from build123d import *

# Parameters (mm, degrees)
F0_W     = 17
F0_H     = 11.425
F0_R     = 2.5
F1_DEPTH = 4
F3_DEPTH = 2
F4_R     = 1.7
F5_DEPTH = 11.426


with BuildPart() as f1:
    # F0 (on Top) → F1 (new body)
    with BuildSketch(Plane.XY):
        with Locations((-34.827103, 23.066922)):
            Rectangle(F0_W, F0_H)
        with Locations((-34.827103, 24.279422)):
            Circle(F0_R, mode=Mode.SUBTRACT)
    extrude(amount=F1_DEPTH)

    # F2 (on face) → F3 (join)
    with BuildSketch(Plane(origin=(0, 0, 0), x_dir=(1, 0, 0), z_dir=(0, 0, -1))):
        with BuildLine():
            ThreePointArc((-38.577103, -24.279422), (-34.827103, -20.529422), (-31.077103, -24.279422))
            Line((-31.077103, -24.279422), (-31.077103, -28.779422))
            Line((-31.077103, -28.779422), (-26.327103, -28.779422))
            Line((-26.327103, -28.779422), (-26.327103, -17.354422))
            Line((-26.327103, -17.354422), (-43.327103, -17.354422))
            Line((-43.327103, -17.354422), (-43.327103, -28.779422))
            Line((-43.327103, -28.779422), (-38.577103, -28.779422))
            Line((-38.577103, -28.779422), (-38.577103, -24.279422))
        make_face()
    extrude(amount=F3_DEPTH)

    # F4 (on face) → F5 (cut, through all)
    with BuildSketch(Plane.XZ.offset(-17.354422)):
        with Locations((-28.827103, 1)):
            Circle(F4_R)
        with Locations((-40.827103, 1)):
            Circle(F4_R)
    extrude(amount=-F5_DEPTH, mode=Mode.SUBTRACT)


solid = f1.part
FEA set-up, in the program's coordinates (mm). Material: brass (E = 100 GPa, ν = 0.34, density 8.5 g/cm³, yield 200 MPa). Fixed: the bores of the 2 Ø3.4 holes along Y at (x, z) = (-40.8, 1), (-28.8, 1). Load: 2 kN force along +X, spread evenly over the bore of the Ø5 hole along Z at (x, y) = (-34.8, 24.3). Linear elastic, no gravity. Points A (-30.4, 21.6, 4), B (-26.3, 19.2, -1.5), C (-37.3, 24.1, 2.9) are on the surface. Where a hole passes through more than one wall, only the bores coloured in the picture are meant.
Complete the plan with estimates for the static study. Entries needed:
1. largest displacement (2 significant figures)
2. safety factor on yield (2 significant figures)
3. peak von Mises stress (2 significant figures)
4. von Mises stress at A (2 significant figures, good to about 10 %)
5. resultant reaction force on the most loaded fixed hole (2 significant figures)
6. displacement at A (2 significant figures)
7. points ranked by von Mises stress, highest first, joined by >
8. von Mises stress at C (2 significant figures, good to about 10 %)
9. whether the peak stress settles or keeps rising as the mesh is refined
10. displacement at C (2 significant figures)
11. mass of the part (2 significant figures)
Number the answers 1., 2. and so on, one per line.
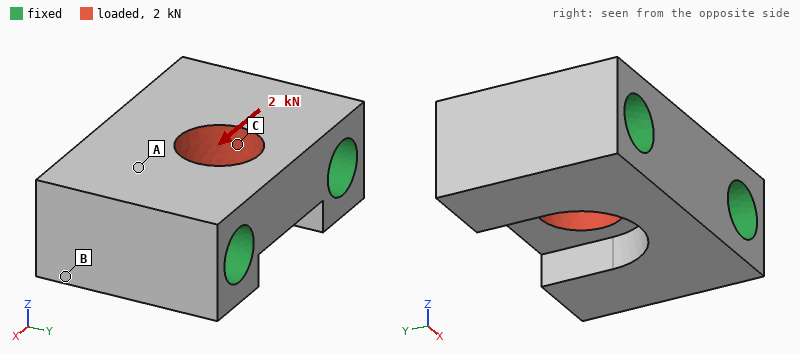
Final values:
1. 1.5 µm
2. 3.6
3. 56 MPa
4. 18 MPa
5. 1.0 kN
6. 0.44 µm
7. C > A > B
8. 32 MPa
9. settles
10. 1.0 µm
11. 6.5 g
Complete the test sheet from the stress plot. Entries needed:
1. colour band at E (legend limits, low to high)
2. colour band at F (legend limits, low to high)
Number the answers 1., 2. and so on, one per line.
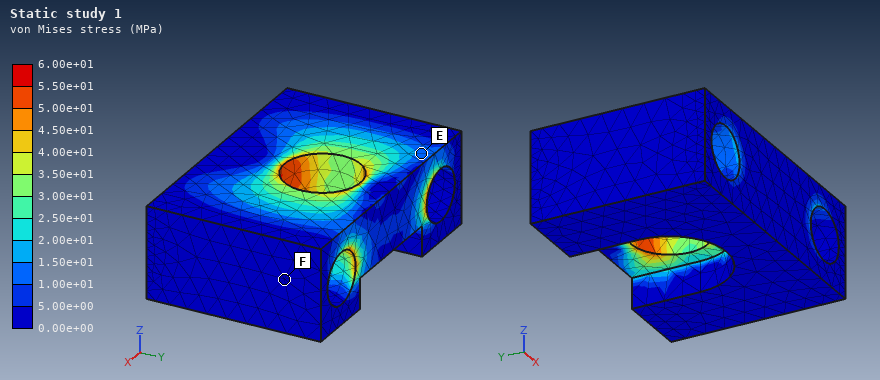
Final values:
1. 1.00e+01 to 1.50e+01 MPa
2. 0.00e+00 to 5.00e+00 MPa
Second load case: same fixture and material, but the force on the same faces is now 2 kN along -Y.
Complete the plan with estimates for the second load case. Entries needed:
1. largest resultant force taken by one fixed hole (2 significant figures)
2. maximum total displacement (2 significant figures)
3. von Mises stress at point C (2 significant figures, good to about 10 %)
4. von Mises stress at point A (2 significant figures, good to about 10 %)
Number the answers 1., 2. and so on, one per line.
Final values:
1. 1.0 kN
2. 4.3 µm
3. 61 MPa
4. 24 MPa
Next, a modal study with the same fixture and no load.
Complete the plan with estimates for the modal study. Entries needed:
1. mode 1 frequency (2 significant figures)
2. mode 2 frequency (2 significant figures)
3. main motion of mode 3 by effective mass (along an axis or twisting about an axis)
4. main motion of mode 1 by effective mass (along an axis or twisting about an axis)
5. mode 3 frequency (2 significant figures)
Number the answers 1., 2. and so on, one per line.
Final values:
1. 93 kHz
2. 98 kHz
3. along Y
4. along Z
5. 110 kHz
